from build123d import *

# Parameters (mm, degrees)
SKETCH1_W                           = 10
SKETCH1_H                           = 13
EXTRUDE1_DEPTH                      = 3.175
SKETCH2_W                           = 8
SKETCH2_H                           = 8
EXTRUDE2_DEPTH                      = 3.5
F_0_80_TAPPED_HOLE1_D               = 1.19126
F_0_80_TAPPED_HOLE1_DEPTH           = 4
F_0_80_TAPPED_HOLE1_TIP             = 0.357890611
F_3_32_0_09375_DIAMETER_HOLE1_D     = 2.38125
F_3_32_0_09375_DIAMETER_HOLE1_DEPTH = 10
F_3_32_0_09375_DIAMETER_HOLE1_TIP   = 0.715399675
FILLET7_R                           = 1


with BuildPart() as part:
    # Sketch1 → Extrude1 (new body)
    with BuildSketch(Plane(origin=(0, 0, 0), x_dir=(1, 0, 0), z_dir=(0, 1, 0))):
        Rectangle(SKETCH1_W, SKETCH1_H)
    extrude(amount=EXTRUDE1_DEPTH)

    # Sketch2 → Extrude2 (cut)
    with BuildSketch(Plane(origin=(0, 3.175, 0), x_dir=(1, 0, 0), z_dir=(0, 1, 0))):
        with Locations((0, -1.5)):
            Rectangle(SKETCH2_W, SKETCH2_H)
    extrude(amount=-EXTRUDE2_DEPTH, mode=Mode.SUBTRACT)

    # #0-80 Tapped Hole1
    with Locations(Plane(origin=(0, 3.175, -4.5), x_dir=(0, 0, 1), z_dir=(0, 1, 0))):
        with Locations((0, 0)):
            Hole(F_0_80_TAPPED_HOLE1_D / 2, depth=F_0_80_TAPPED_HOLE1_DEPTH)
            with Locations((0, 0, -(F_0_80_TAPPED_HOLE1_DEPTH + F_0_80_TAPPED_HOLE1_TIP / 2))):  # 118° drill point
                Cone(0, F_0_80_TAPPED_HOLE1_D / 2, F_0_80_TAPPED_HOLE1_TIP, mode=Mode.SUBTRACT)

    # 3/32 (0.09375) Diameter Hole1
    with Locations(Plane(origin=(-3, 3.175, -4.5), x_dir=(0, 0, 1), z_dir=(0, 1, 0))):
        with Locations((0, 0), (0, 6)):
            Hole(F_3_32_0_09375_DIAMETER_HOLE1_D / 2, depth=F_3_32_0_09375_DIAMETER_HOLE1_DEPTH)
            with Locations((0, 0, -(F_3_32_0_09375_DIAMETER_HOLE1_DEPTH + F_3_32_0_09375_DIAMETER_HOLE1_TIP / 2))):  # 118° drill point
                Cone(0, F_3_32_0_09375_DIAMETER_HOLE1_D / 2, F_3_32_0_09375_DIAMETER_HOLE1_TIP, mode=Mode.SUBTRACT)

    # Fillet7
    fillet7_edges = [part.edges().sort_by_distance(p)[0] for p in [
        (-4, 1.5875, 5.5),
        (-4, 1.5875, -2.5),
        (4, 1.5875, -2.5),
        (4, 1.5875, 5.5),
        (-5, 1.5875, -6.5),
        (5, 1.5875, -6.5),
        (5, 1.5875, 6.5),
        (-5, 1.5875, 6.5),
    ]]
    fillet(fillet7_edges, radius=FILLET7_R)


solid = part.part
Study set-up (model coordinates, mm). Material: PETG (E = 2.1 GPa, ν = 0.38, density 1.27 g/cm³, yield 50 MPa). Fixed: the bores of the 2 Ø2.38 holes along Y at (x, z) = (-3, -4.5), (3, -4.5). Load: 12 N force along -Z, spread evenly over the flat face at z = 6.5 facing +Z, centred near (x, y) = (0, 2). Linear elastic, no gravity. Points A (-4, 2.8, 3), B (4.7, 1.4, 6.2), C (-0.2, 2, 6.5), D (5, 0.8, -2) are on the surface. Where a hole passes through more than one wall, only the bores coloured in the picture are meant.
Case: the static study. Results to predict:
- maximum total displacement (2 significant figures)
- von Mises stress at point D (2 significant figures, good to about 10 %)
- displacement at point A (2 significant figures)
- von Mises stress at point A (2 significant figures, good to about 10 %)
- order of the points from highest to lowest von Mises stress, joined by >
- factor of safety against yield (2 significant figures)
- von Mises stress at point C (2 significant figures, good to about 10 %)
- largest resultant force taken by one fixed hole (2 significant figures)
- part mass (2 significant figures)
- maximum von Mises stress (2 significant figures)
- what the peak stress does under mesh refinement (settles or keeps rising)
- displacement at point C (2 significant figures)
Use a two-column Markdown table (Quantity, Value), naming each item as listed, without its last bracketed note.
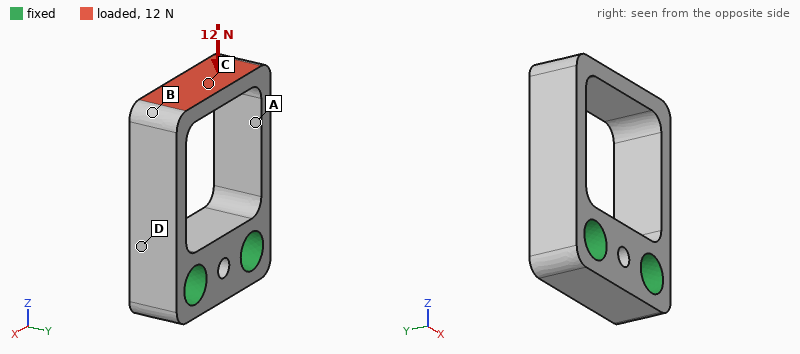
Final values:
| Quantity | Value |
|---|---|
| maximum total displacement | 99 µm |
| von Mises stress at point D | 6.1 MPa |
| displacement at point A | 41 µm |
| von Mises stress at point A | 9.1 MPa |
| order of the points from highest to lowest von Mises stress, joined by > | C > A > D > B |
| factor of safety against yield | 3.3 |
| von Mises stress at point C | 13 MPa |
| largest resultant force taken by one fixed hole | 6.1 N |
| part mass | 0.23 g |
| maximum von Mises stress | 15 MPa |
| what the peak stress does under mesh refinement | settles |
| displacement at point C | 94 µm |
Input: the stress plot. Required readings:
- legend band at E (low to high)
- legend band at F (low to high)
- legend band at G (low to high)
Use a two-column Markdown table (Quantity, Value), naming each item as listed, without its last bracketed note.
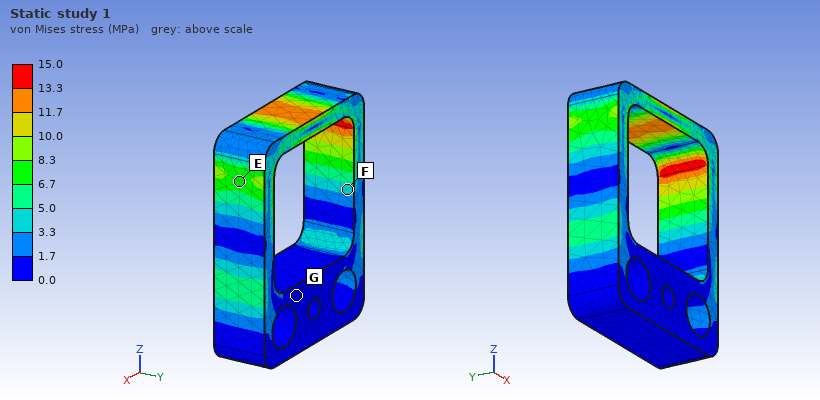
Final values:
| Quantity | Value |
|---|---|
| legend band at E | 6.7 to 8.3 MPa |
| legend band at F | 3.3 to 5.0 MPa |
| legend band at G | 0.0 to 1.7 MPa |
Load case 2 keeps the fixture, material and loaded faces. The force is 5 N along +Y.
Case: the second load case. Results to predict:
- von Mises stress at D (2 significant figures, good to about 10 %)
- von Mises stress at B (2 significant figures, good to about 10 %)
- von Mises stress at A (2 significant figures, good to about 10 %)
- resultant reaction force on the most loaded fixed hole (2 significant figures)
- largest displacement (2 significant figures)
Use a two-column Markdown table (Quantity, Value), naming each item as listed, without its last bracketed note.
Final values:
| Quantity | Value |
|---|---|
| von Mises stress at D | 5.2 MPa |
| von Mises stress at B | 2.5 MPa |
| von Mises stress at A | 4.3 MPa |
| resultant reaction force on the most loaded fixed hole | 2.5 N |
| largest displacement | 0.17 mm |
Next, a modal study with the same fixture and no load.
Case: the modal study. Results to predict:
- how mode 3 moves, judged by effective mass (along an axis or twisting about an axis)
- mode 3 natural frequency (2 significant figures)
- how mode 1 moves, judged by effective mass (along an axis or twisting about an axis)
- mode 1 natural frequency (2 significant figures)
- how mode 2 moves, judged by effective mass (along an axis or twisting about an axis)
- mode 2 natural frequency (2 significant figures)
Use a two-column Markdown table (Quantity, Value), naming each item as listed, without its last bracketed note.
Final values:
| Quantity | Value |
|---|---|
| how mode 3 moves, judged by effective mass | twisting about Z |
| mode 3 natural frequency | 6400 Hz |
| how mode 1 moves, judged by effective mass | along X |
| mode 1 natural frequency | 2800 Hz |
| how mode 2 moves, judged by effective mass | along Y |
| mode 2 natural frequency | 4000 Hz |
